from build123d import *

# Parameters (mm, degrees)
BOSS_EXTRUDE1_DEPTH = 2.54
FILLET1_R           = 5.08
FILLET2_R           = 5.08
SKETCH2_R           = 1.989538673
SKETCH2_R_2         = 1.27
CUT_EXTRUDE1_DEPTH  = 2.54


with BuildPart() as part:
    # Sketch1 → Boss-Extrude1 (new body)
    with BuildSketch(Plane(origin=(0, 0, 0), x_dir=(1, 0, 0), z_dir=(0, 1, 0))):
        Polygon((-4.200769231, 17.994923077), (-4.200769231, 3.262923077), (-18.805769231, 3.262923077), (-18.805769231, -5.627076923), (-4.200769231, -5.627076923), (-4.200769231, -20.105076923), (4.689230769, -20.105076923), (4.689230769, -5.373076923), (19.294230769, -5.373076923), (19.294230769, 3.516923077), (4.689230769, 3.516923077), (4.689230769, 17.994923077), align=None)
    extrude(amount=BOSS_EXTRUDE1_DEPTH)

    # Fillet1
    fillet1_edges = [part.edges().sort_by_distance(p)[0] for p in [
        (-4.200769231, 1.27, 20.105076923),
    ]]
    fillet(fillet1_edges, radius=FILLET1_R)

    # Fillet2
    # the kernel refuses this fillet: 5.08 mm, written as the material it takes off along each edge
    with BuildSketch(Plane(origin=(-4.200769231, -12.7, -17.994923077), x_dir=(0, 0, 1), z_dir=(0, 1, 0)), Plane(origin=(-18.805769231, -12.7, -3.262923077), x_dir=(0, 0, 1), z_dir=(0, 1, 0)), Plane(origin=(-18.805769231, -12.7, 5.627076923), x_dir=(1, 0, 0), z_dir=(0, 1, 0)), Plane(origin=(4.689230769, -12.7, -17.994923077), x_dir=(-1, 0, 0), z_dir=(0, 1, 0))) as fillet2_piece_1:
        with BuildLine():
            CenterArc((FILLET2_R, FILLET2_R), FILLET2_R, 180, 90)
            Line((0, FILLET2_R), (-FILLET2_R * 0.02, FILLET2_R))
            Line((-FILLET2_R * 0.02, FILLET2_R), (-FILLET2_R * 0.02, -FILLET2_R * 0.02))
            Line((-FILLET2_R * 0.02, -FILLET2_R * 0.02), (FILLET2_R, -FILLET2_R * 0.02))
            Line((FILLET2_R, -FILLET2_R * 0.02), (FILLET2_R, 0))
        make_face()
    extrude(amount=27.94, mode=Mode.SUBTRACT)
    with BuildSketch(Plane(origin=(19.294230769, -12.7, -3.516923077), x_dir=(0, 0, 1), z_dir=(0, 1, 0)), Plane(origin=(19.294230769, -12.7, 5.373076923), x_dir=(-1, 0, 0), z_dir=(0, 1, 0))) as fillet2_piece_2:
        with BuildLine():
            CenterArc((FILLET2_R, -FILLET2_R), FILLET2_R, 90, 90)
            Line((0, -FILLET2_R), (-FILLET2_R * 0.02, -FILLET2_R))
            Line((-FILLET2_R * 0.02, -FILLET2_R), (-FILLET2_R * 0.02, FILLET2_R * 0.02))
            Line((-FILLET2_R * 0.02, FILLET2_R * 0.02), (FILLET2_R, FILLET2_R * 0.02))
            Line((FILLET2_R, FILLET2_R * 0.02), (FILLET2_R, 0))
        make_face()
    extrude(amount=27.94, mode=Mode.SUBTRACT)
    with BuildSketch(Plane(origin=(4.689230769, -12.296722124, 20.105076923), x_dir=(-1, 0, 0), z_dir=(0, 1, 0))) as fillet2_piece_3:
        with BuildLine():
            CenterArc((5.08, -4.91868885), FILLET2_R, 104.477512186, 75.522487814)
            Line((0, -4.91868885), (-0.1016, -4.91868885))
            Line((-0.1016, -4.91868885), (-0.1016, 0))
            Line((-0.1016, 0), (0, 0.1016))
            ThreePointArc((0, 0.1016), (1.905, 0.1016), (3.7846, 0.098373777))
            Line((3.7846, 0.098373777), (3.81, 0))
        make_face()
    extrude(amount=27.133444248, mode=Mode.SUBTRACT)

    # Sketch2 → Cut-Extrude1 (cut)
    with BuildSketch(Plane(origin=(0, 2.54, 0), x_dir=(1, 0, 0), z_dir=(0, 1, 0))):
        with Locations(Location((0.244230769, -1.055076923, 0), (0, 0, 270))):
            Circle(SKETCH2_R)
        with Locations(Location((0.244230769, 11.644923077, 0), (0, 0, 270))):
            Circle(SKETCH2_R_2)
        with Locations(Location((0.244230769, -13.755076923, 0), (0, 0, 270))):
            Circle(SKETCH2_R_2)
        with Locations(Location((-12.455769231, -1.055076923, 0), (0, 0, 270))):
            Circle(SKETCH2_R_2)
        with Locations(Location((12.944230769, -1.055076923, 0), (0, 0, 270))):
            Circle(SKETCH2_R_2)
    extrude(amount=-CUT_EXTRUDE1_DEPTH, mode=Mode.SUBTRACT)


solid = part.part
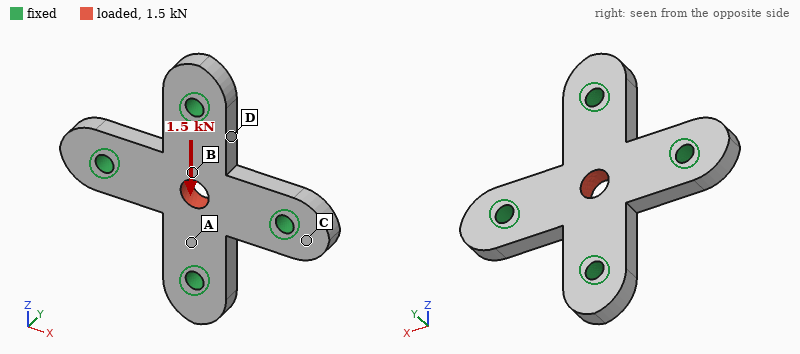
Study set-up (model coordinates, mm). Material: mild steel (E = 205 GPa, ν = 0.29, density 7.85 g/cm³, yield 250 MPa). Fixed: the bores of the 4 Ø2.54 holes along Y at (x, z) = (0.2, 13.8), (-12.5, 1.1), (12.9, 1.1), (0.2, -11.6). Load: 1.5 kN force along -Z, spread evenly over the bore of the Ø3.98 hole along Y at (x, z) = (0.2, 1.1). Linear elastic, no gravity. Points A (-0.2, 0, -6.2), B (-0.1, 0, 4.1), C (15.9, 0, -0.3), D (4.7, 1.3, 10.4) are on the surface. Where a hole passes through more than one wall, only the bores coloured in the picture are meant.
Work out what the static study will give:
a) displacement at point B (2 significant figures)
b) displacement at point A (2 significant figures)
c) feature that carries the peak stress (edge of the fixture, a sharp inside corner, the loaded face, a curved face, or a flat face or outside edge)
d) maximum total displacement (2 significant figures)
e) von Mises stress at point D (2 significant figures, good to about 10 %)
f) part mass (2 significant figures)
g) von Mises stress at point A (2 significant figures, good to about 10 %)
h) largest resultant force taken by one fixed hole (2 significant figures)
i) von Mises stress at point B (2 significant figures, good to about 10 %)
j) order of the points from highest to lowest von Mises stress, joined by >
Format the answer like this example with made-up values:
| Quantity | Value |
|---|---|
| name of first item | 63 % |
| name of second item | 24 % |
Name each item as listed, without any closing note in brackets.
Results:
| Quantity | Value |
|---|---|
| displacement at point B | 1.7 µm |
| displacement at point A | 0.89 µm |
| feature that carries the peak stress | the loaded face |
| maximum total displacement | 2.1 µm |
| von Mises stress at point D | 20 MPa |
| part mass | 10 g |
| von Mises stress at point A | 38 MPa |
| largest resultant force taken by one fixed hole | 660 N |
| von Mises stress at point B | 51 MPa |
| order of the points from highest to lowest von Mises stress, joined by > | B > A > D > C |
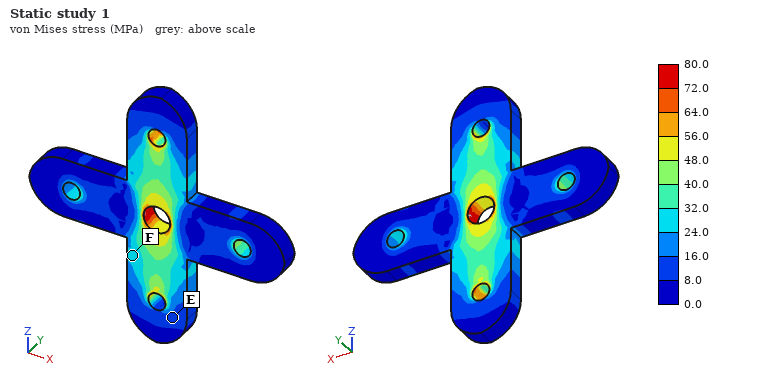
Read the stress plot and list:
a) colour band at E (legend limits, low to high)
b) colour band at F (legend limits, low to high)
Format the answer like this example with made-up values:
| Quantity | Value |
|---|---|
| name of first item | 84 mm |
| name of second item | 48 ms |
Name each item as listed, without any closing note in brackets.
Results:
| Quantity | Value |
|---|---|
| colour band at E | 8.0 to 16.0 MPa |
| colour band at F | 24.0 to 32.0 MPa |
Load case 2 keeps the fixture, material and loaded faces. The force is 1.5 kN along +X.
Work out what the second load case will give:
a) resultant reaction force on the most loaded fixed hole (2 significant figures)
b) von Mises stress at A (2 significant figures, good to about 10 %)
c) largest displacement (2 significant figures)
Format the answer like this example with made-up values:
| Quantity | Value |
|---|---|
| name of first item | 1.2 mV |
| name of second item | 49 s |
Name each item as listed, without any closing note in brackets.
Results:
| Quantity | Value |
|---|---|
| resultant reaction force on the most loaded fixed hole | 660 N |
| von Mises stress at A | 8.2 MPa |
| largest displacement | 2.1 µm |
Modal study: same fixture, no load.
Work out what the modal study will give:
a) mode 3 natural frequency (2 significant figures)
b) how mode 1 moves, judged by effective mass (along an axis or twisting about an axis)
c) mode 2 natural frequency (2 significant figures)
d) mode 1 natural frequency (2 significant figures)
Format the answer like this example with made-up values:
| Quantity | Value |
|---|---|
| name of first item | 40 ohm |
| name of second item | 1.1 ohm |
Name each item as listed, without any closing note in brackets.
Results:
| Quantity | Value |
|---|---|
| mode 3 natural frequency | 52 kHz |
| how mode 1 moves, judged by effective mass | along Y |
| mode 2 natural frequency | 52 kHz |
| mode 1 natural frequency | 29 kHz |
